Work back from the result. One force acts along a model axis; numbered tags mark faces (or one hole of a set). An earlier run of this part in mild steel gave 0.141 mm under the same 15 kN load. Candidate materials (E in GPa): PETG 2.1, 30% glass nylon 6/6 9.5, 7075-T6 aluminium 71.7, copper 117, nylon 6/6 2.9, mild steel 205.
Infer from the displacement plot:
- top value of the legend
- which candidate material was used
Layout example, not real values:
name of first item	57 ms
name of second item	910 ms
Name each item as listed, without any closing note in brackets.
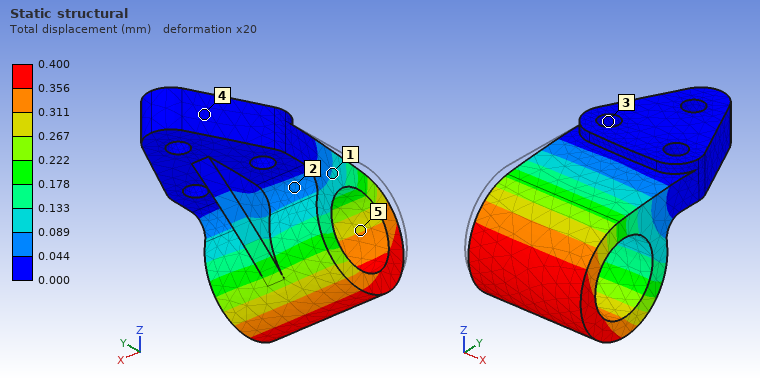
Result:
top value of the legend	0.400 mm
which candidate material was used	7075-T6 aluminium
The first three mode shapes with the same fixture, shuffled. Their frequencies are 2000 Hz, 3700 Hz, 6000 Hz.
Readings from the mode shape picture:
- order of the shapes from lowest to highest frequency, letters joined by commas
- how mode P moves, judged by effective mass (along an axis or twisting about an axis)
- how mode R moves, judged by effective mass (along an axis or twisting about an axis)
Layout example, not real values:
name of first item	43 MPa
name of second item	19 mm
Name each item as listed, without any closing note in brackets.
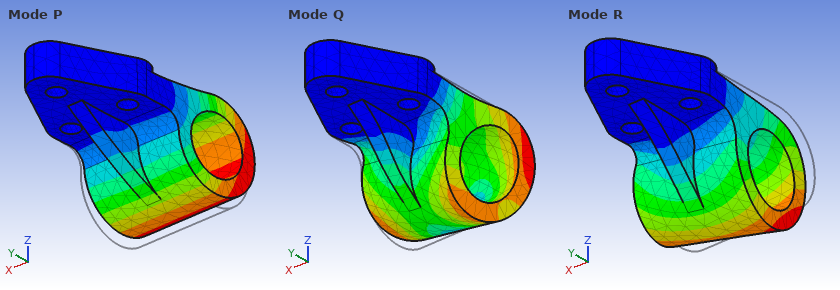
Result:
order of the shapes from lowest to highest frequency, letters joined by commas	P, R, Q
how mode P moves, judged by effective mass	along Z
how mode R moves, judged by effective mass	along X
